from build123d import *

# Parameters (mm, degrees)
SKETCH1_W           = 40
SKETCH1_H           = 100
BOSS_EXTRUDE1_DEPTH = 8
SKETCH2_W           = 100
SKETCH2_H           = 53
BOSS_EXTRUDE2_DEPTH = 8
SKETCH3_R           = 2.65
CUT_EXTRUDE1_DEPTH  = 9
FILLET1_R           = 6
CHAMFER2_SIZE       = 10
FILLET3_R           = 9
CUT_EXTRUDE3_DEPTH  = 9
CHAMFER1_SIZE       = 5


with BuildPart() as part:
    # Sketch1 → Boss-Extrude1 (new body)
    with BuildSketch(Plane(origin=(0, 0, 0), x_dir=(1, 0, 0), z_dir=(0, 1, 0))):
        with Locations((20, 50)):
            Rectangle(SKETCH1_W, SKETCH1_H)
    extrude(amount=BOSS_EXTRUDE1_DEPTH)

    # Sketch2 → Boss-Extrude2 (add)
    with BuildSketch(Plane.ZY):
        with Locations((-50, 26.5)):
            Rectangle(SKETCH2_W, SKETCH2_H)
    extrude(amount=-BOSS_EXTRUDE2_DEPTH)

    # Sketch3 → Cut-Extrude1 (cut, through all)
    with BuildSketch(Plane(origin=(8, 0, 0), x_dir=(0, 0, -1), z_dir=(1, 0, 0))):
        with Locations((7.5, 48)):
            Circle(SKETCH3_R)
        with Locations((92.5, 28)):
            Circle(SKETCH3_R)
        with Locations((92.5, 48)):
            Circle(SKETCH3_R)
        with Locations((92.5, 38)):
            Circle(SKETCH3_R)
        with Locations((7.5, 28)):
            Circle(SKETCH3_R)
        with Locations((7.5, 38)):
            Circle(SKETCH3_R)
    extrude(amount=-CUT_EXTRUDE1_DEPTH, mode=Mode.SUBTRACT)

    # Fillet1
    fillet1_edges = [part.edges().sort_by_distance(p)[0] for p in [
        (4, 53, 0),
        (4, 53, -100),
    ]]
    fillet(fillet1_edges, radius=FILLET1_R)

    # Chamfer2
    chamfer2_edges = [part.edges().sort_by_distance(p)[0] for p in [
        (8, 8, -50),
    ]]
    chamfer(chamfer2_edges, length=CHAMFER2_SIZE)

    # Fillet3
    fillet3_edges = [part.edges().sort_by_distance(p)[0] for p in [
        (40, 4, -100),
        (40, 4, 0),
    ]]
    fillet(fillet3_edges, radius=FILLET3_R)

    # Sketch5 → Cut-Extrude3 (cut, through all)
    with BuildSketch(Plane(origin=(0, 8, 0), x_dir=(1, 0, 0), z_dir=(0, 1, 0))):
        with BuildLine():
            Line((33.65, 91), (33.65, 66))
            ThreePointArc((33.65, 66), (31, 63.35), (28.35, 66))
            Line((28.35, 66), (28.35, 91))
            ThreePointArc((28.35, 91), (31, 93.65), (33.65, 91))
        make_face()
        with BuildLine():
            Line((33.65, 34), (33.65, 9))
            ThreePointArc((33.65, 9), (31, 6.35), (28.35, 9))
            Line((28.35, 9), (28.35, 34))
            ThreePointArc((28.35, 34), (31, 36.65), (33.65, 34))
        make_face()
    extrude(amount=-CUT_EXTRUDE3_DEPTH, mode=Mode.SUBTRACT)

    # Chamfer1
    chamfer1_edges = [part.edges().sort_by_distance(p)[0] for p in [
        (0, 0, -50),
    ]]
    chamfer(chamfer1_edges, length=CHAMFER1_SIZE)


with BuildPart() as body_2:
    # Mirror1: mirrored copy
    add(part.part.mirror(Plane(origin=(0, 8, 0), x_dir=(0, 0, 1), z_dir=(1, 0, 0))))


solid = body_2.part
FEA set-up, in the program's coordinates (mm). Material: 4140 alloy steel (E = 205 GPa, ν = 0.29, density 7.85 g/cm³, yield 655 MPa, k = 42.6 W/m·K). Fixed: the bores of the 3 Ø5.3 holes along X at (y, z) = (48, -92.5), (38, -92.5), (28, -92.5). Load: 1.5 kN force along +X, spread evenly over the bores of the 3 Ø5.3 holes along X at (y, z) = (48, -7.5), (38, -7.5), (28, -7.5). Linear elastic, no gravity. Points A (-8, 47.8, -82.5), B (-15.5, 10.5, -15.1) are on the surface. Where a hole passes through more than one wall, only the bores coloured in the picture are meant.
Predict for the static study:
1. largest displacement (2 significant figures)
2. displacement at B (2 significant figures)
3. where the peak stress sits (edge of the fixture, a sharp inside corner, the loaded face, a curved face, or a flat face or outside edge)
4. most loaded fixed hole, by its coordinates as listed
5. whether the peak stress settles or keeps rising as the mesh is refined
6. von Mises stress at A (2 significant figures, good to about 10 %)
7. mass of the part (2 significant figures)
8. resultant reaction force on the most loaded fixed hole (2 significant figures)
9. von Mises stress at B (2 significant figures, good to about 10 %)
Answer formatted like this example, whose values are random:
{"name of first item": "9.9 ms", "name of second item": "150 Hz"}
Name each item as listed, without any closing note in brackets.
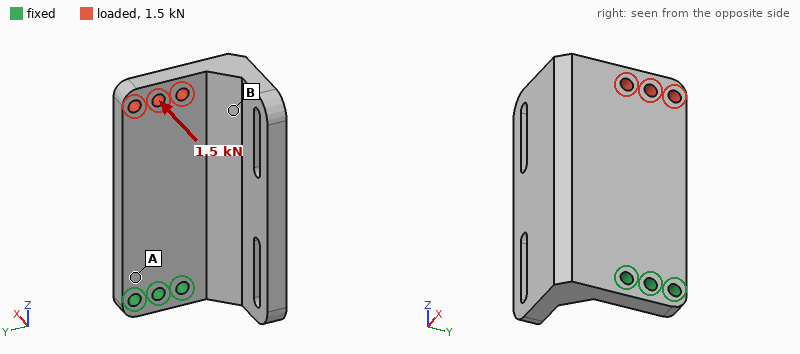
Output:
{"largest displacement": "0.43 mm", "displacement at B": "0.31 mm", "where the peak stress sits": "edge of the fixture", "most loaded fixed hole, by its coordinates as listed": "(38, -92.5)", "whether the peak stress settles or keeps rising as the mesh is refined": "keeps rising", "von Mises stress at A": "170 MPa", "mass of the part": "530 g", "resultant reaction force on the most loaded fixed hole": "1.5 kN", "von Mises stress at B": "36 MPa"}
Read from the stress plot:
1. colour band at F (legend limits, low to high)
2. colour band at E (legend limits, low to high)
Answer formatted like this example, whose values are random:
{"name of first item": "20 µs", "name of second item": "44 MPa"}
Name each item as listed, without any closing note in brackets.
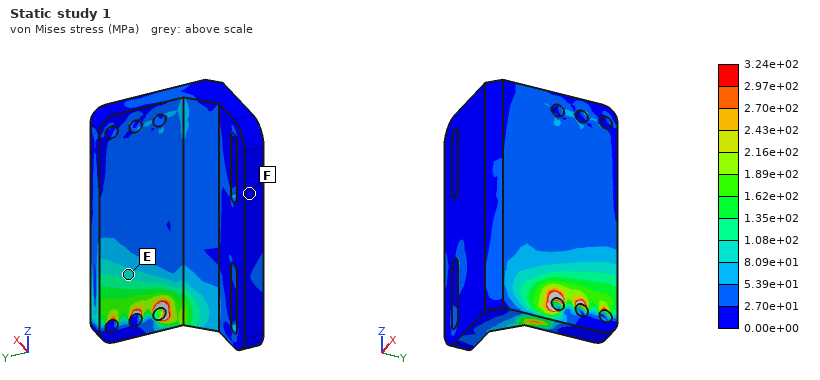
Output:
{"colour band at F": "0.00e+00 to 2.70e+01 MPa", "colour band at E": "8.09e+01 to 1.08e+02 MPa"}
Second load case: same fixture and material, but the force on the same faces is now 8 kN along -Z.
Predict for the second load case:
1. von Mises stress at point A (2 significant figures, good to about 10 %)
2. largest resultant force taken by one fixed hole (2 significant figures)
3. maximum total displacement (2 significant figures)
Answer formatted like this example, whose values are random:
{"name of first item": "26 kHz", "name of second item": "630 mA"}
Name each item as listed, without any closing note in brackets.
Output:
{"von Mises stress at point A": "38 MPa", "largest resultant force taken by one fixed hole": "3.0 kN", "maximum total displacement": "22 µm"}
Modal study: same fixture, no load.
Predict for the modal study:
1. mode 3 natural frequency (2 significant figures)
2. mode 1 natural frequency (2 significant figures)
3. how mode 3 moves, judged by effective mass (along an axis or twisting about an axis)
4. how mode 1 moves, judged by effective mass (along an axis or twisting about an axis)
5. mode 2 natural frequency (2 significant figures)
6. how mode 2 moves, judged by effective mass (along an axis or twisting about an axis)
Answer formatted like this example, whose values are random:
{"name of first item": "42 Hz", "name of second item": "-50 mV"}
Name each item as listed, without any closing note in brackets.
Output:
{"mode 3 natural frequency": "2300 Hz", "mode 1 natural frequency": "710 Hz", "how mode 3 moves, judged by effective mass": "along Y", "how mode 1 moves, judged by effective mass": "along X", "mode 2 natural frequency": "1700 Hz", "how mode 2 moves, judged by effective mass": "along Y"}
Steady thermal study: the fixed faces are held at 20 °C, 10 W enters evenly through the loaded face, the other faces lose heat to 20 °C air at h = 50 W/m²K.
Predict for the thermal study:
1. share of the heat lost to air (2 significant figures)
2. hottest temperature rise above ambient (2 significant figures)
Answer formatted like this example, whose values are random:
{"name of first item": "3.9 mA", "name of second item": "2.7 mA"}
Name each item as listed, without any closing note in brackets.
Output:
{"share of the heat lost to air": "72 %", "hottest temperature rise above ambient": "29 K"}
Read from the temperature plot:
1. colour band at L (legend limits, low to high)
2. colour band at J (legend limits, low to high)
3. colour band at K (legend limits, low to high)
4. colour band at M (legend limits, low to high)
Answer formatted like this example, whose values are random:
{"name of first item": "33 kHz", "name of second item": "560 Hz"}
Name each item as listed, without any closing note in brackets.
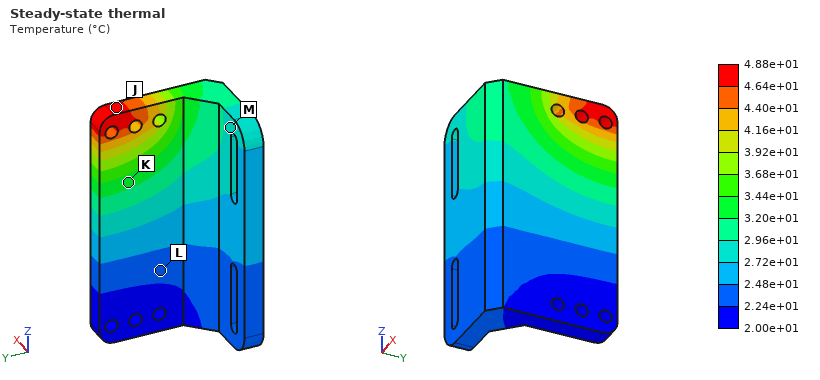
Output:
{"colour band at L": "2.24e+01 to 2.48e+01 °C", "colour band at J": "4.64e+01 to 4.88e+01 °C", "colour band at K": "3.20e+01 to 3.44e+01 °C", "colour band at M": "2.72e+01 to 2.96e+01 °C"}
